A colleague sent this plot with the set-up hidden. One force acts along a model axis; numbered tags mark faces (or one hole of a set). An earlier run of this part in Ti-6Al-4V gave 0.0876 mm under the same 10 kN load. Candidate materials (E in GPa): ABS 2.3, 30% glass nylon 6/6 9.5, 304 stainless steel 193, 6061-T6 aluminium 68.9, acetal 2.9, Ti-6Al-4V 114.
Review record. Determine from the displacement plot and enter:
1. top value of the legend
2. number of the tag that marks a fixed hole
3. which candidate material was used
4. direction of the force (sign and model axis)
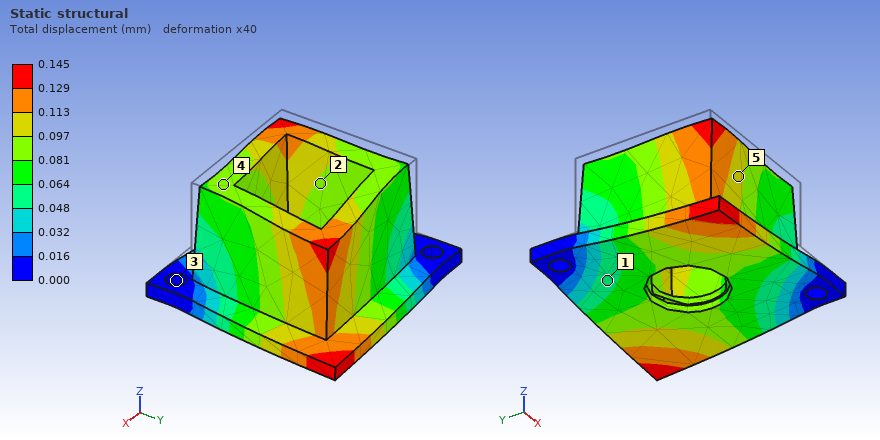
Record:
0.145 mm
3
6061-T6 aluminium
-Z
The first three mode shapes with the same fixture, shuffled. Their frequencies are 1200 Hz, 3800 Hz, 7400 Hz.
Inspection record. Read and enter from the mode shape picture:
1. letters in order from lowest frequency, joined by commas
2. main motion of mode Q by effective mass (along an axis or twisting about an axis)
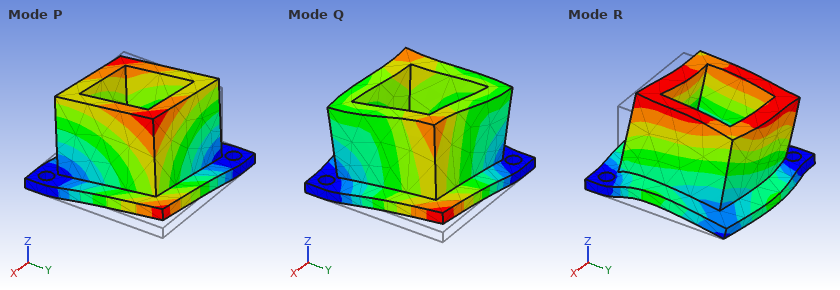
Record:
P, Q, R
along Z
